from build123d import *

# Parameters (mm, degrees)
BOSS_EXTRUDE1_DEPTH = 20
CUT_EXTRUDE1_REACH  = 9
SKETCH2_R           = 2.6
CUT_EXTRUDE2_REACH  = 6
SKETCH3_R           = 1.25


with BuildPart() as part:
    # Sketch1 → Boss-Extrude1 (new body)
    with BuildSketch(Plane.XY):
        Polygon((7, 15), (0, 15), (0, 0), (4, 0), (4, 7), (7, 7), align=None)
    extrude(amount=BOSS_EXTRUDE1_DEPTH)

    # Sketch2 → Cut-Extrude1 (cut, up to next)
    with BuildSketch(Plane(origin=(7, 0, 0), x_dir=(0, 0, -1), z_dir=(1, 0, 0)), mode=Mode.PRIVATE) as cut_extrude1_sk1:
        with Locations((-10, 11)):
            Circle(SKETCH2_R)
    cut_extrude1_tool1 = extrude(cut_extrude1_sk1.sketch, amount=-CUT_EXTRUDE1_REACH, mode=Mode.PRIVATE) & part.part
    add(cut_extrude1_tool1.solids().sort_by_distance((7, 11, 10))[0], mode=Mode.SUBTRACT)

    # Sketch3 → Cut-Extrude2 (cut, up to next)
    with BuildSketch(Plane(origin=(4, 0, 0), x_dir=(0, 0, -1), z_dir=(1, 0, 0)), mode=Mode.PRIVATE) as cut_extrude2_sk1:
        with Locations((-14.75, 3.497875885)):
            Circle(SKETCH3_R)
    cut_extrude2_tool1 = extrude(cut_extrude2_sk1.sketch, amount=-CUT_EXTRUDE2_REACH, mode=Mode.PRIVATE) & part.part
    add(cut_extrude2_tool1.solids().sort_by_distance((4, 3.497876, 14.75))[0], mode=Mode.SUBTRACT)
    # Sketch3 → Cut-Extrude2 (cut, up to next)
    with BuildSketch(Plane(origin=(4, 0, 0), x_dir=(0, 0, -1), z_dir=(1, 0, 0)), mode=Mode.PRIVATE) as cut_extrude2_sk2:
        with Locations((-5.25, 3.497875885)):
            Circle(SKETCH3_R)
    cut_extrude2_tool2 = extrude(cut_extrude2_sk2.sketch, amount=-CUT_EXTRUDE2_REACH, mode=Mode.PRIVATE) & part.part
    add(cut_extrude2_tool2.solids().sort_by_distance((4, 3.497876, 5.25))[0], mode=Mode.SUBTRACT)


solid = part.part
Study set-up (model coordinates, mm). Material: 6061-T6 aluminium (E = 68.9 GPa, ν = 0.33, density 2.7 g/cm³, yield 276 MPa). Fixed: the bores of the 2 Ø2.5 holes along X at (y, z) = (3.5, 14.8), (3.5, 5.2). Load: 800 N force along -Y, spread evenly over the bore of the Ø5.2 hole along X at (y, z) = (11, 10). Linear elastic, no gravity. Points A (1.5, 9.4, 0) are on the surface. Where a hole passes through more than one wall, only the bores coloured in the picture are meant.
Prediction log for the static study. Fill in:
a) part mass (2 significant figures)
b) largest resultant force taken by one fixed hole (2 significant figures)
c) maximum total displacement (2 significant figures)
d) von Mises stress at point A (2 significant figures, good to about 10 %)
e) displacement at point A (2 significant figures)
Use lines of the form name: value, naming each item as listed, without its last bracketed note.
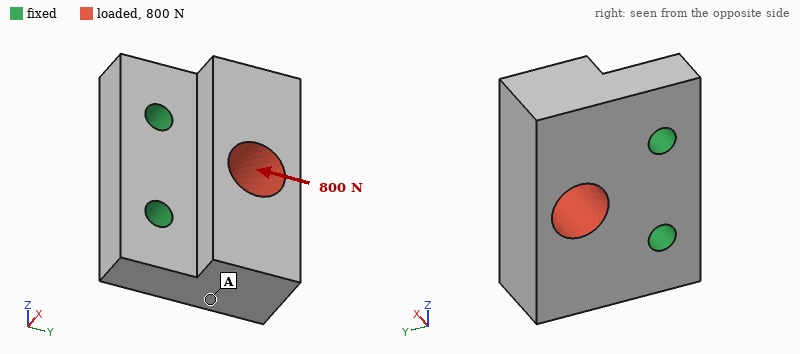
part mass: 4.0 g
largest resultant force taken by one fixed hole: 410 N
maximum total displacement: 11 µm
von Mises stress at point A: 7.6 MPa
displacement at point A: 2.7 µm
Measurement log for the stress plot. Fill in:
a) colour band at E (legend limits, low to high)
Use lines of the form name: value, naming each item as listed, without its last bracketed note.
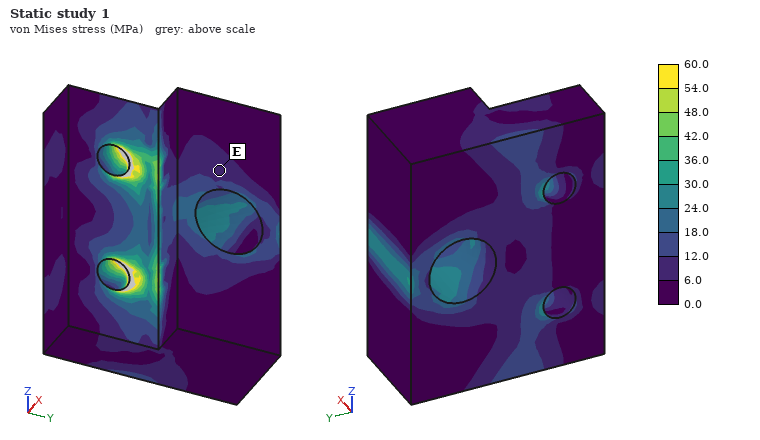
colour band at E: 6.0 to 12.0 MPa
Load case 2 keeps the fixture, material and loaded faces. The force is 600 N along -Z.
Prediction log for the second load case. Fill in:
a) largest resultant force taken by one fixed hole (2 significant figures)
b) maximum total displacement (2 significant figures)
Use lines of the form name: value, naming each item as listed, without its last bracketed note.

largest resultant force taken by one fixed hole: 470 N
maximum total displacement: 7.2 µm
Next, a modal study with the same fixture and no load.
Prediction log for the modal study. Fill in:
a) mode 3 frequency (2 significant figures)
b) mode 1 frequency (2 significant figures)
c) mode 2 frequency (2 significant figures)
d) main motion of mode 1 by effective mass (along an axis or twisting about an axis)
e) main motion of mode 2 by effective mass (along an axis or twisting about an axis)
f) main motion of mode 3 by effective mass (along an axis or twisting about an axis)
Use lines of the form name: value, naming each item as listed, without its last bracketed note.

mode 3 frequency: 32 kHz
mode 1 frequency: 17 kHz
mode 2 frequency: 27 kHz
main motion of mode 1 by effective mass: along X
main motion of mode 2 by effective mass: twisting about Y
main motion of mode 3 by effective mass: along Z
